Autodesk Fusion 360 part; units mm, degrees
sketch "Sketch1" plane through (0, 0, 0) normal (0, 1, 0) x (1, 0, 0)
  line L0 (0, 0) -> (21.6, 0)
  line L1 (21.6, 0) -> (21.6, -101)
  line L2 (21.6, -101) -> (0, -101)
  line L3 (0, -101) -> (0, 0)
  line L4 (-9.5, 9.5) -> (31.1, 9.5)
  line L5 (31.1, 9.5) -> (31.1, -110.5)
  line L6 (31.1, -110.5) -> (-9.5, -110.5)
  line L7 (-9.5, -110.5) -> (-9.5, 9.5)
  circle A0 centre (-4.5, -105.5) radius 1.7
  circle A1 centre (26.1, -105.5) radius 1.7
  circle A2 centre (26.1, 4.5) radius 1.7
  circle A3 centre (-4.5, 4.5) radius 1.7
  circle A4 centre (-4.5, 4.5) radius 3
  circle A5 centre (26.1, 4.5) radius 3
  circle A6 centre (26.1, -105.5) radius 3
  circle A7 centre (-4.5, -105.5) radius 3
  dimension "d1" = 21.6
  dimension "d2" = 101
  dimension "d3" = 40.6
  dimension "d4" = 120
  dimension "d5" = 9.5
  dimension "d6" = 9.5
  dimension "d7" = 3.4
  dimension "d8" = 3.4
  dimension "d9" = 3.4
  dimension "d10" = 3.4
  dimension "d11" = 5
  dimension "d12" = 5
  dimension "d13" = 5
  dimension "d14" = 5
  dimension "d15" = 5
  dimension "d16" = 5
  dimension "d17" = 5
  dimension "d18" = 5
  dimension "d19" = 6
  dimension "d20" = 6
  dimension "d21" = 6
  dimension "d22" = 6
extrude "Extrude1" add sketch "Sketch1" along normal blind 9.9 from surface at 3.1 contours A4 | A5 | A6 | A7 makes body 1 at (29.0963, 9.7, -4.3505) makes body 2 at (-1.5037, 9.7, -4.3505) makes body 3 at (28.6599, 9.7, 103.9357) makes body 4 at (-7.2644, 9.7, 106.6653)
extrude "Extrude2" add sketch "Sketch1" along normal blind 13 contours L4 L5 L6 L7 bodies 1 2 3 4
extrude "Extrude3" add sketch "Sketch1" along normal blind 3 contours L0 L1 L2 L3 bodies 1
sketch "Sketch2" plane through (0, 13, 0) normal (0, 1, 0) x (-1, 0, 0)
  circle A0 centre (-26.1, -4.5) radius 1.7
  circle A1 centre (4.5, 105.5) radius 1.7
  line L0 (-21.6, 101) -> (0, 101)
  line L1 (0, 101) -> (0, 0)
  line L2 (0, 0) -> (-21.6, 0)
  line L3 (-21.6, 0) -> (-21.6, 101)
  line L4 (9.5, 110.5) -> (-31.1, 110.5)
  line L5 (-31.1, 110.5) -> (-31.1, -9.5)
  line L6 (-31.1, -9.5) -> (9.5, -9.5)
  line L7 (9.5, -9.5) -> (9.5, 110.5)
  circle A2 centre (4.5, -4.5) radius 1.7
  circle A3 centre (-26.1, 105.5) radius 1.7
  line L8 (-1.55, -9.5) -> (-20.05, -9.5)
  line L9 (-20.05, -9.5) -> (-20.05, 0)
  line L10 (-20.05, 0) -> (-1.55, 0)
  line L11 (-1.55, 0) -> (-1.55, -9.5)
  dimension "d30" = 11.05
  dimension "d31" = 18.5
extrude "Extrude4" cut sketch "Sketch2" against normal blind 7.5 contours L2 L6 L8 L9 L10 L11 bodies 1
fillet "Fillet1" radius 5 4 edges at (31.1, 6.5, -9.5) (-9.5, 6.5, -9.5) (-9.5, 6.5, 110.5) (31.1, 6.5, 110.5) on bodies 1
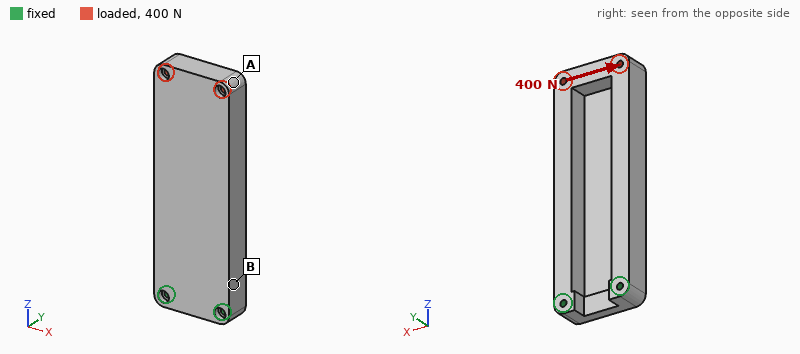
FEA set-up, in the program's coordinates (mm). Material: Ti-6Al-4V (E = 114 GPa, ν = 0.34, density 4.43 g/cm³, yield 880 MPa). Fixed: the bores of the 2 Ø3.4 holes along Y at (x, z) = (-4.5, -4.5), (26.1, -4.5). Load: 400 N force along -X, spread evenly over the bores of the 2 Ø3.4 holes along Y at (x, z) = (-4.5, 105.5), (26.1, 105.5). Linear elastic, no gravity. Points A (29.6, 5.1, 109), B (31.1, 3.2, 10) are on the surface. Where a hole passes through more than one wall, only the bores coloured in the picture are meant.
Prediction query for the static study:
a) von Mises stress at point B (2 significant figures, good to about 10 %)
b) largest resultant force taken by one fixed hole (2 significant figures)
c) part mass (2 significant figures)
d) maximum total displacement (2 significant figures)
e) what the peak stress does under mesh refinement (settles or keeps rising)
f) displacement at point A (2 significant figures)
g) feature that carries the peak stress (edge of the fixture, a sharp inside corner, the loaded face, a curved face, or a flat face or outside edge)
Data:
17 MPa
1.3 kN
170 g
69 µm
keeps rising
58 µm
edge of the fixture
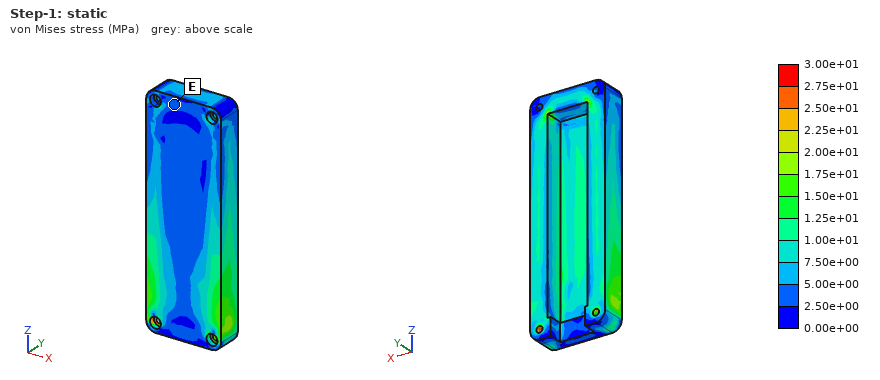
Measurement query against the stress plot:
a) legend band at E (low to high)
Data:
2.50e+00 to 5.00e+00 MPa
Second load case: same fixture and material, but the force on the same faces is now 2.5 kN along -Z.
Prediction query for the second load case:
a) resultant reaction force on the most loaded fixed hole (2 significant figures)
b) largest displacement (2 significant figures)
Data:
1.3 kN
74 µm
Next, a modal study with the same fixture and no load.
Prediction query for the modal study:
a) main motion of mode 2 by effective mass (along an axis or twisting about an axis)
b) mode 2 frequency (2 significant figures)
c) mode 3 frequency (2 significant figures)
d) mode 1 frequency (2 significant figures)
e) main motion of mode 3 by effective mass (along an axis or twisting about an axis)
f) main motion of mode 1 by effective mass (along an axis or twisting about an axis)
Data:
along X
1700 Hz
2900 Hz
700 Hz
along X
along Y
